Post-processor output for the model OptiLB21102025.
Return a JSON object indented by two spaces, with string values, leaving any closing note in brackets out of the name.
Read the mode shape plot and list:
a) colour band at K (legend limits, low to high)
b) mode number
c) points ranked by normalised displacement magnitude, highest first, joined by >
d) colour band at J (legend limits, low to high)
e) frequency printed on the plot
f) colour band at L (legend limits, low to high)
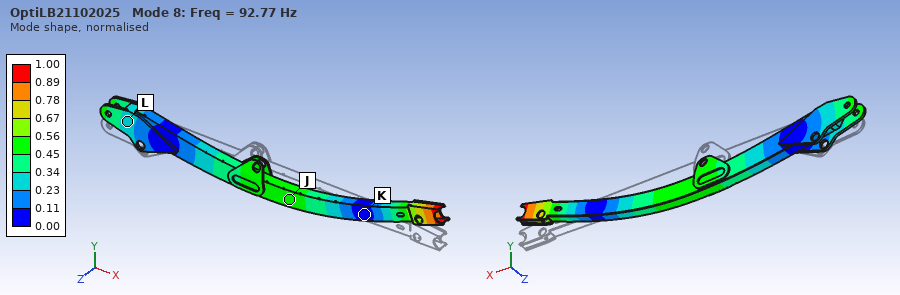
{
  "colour band at K": "0.00 to 0.11",
  "mode number": "8",
  "points ranked by normalised displacement magnitude, highest first, joined by >": "J > L > K",
  "colour band at J": "0.45 to 0.56",
  "frequency printed on the plot": "92.77 Hz",
  "colour band at L": "0.23 to 0.34"
}
